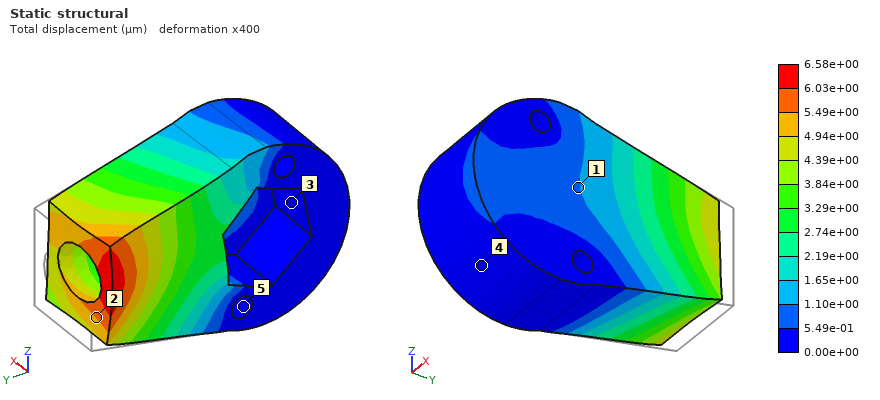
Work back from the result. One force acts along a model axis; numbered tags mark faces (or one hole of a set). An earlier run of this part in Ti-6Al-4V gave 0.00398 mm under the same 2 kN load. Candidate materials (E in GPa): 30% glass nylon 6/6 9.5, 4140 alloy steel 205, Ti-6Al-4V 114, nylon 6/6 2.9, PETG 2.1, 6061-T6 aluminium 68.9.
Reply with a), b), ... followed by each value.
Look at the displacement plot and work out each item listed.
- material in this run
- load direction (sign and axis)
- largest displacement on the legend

a) 6061-T6 aluminium
b) -Y
c) 6.58e+00 µm
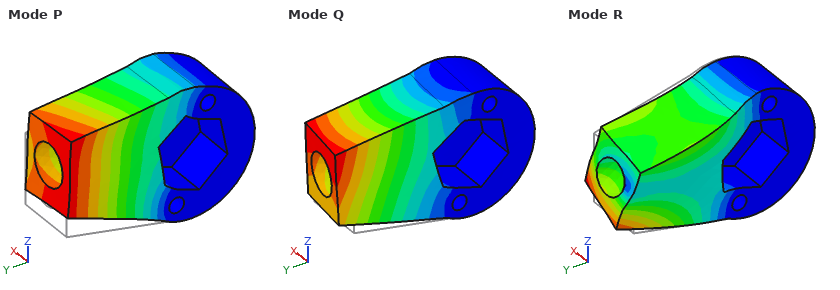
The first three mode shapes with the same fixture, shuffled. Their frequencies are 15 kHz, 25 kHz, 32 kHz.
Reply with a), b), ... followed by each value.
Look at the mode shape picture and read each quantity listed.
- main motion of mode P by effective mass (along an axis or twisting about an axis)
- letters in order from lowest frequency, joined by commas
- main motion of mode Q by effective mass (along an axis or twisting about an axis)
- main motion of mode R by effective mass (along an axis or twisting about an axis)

a) along Z
b) Q, P, R
c) along X
d) twisting about Y
